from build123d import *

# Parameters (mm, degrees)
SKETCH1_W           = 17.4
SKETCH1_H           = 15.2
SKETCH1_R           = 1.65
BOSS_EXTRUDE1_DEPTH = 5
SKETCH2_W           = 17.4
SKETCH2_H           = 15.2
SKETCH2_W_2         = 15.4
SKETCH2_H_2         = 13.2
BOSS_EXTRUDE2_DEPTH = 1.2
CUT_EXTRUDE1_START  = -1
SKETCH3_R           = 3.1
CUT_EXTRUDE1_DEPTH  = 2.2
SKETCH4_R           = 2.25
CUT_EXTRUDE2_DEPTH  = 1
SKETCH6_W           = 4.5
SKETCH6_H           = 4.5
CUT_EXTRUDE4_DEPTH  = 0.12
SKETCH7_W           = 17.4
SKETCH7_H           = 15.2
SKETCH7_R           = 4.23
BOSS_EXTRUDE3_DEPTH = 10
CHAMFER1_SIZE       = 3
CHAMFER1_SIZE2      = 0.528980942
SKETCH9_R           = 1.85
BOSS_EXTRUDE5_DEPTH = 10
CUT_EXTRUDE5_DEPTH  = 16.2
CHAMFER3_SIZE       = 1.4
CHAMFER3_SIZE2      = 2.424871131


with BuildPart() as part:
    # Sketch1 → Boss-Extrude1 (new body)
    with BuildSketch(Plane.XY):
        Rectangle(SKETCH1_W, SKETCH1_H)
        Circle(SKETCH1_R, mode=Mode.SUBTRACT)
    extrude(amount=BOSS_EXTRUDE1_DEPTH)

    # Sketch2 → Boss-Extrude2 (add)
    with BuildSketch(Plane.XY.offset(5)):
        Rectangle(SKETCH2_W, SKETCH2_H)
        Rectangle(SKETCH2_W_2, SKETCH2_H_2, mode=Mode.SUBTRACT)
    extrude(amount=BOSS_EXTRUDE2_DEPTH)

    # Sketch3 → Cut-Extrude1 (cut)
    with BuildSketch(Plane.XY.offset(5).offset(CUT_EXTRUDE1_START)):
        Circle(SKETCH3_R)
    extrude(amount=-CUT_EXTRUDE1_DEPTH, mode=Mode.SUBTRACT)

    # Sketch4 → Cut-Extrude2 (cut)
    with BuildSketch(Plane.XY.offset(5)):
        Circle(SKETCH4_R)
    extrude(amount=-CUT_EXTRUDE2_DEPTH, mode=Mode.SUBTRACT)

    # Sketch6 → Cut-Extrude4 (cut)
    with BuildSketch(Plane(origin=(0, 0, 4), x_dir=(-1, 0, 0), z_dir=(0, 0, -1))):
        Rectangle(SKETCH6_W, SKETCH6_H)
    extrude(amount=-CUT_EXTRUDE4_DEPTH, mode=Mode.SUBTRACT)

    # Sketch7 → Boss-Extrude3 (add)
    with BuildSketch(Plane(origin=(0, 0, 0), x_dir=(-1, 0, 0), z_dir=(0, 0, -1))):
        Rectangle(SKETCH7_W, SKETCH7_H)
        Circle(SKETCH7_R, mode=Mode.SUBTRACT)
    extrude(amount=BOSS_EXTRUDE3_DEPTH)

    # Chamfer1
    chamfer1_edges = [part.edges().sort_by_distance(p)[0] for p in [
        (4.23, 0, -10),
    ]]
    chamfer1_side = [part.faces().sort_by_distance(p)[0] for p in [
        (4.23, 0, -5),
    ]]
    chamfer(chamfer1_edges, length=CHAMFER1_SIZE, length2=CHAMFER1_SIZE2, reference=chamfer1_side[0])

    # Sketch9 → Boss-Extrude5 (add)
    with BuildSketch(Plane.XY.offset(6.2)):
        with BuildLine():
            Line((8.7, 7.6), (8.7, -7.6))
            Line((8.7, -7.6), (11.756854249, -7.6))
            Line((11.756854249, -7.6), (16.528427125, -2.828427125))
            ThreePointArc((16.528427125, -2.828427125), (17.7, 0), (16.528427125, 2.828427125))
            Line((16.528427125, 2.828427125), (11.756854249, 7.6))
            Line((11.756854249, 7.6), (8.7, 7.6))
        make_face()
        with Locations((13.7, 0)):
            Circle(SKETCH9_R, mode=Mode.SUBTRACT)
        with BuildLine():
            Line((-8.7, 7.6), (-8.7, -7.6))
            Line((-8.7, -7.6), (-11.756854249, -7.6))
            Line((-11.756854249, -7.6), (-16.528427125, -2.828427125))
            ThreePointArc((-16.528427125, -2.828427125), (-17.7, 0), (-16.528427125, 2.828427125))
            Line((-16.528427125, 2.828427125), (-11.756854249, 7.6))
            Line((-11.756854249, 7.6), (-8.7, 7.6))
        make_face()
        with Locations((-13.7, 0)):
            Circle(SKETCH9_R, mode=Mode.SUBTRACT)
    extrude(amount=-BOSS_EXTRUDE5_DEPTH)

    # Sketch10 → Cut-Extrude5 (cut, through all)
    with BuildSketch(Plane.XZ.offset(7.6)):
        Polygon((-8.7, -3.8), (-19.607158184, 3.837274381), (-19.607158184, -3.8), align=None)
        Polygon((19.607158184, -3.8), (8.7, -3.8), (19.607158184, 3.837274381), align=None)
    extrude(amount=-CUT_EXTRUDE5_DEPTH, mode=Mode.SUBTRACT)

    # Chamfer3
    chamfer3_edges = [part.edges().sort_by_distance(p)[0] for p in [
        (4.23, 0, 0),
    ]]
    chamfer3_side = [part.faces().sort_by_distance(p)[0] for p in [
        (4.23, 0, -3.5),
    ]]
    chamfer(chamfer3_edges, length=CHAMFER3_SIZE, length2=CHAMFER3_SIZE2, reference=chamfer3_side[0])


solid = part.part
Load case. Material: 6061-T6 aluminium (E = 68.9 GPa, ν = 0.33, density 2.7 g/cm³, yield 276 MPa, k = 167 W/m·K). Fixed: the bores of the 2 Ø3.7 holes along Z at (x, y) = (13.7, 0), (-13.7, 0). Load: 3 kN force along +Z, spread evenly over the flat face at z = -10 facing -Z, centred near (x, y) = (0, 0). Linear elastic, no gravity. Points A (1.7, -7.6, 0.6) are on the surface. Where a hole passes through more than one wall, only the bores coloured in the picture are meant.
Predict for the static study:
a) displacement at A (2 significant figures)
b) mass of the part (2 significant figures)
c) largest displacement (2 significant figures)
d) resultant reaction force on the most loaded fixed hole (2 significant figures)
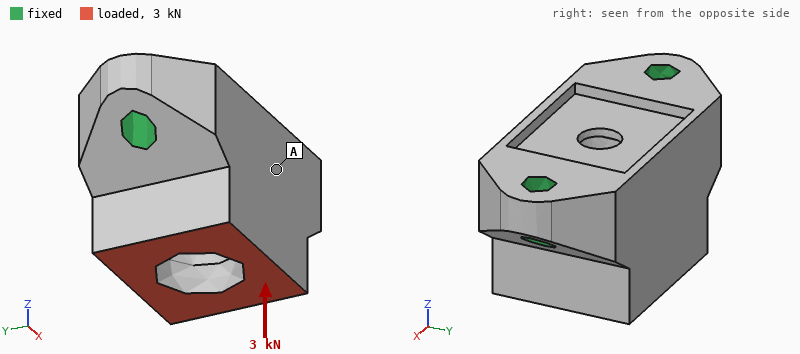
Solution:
7.5 µm
13 g
8.9 µm
1.6 kN
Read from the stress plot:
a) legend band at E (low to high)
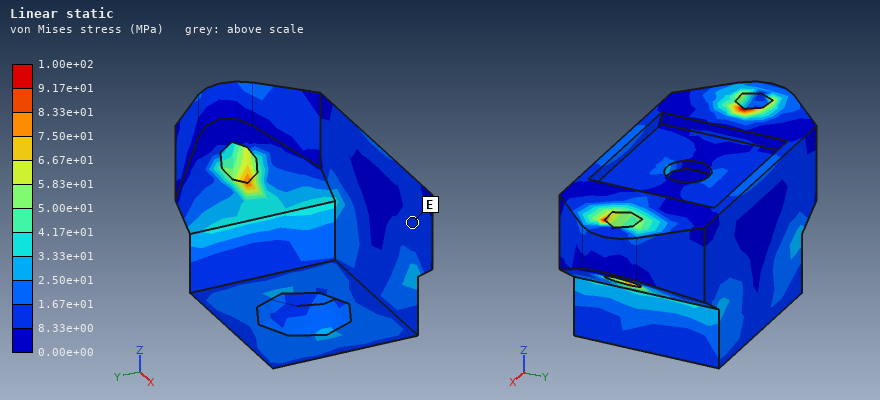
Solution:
8.33e+00 to 1.67e+01 MPa
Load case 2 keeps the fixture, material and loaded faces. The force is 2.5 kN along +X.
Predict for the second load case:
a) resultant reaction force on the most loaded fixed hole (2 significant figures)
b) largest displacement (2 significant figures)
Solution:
1.7 kN
14 µm
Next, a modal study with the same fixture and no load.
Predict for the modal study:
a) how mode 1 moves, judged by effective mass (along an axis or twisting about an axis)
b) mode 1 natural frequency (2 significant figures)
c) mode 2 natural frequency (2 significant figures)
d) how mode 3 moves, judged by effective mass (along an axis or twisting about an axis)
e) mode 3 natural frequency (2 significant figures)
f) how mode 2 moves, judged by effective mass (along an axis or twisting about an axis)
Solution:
along Y
21 kHz
34 kHz
along Y
43 kHz
along Z
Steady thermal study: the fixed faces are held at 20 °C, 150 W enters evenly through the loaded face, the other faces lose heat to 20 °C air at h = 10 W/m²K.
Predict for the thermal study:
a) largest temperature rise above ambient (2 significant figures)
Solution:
70 K
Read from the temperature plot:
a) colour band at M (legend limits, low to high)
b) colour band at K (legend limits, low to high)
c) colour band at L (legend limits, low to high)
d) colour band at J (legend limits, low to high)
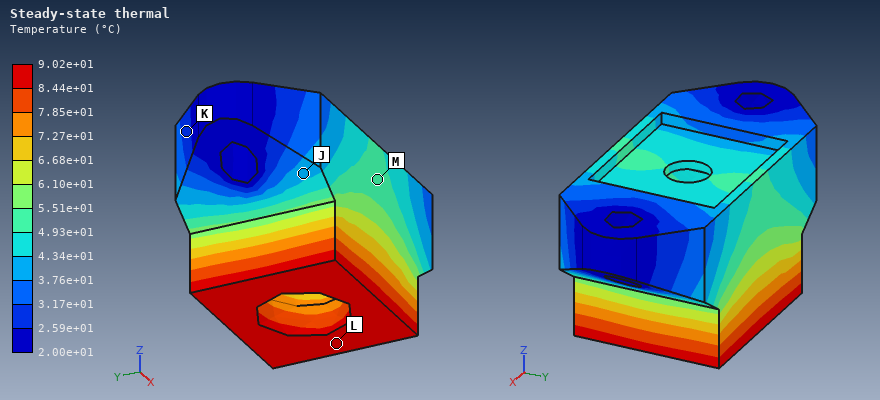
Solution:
4.93e+01 to 5.51e+01 °C
2.59e+01 to 3.17e+01 °C
8.44e+01 to 9.02e+01 °C
3.76e+01 to 4.34e+01 °C
